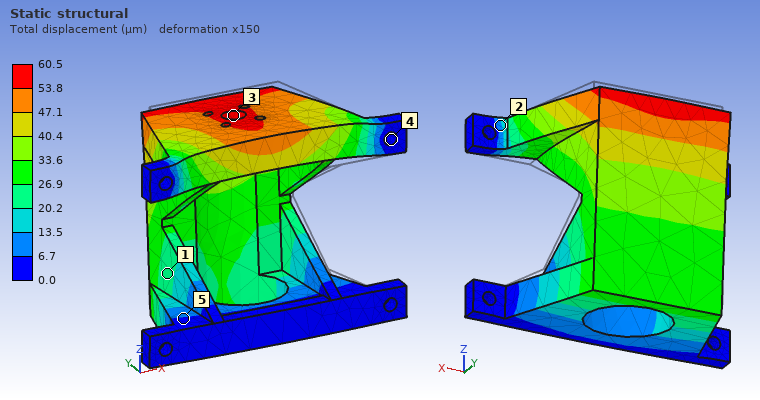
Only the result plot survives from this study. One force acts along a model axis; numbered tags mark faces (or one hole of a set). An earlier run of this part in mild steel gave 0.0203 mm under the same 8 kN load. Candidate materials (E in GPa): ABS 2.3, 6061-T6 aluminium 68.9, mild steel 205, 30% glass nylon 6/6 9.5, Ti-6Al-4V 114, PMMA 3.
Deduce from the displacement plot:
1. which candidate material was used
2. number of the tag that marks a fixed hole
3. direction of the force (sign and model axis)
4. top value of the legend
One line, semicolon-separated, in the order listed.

6061-T6 aluminium; 4; +Y; 60.5 µm
